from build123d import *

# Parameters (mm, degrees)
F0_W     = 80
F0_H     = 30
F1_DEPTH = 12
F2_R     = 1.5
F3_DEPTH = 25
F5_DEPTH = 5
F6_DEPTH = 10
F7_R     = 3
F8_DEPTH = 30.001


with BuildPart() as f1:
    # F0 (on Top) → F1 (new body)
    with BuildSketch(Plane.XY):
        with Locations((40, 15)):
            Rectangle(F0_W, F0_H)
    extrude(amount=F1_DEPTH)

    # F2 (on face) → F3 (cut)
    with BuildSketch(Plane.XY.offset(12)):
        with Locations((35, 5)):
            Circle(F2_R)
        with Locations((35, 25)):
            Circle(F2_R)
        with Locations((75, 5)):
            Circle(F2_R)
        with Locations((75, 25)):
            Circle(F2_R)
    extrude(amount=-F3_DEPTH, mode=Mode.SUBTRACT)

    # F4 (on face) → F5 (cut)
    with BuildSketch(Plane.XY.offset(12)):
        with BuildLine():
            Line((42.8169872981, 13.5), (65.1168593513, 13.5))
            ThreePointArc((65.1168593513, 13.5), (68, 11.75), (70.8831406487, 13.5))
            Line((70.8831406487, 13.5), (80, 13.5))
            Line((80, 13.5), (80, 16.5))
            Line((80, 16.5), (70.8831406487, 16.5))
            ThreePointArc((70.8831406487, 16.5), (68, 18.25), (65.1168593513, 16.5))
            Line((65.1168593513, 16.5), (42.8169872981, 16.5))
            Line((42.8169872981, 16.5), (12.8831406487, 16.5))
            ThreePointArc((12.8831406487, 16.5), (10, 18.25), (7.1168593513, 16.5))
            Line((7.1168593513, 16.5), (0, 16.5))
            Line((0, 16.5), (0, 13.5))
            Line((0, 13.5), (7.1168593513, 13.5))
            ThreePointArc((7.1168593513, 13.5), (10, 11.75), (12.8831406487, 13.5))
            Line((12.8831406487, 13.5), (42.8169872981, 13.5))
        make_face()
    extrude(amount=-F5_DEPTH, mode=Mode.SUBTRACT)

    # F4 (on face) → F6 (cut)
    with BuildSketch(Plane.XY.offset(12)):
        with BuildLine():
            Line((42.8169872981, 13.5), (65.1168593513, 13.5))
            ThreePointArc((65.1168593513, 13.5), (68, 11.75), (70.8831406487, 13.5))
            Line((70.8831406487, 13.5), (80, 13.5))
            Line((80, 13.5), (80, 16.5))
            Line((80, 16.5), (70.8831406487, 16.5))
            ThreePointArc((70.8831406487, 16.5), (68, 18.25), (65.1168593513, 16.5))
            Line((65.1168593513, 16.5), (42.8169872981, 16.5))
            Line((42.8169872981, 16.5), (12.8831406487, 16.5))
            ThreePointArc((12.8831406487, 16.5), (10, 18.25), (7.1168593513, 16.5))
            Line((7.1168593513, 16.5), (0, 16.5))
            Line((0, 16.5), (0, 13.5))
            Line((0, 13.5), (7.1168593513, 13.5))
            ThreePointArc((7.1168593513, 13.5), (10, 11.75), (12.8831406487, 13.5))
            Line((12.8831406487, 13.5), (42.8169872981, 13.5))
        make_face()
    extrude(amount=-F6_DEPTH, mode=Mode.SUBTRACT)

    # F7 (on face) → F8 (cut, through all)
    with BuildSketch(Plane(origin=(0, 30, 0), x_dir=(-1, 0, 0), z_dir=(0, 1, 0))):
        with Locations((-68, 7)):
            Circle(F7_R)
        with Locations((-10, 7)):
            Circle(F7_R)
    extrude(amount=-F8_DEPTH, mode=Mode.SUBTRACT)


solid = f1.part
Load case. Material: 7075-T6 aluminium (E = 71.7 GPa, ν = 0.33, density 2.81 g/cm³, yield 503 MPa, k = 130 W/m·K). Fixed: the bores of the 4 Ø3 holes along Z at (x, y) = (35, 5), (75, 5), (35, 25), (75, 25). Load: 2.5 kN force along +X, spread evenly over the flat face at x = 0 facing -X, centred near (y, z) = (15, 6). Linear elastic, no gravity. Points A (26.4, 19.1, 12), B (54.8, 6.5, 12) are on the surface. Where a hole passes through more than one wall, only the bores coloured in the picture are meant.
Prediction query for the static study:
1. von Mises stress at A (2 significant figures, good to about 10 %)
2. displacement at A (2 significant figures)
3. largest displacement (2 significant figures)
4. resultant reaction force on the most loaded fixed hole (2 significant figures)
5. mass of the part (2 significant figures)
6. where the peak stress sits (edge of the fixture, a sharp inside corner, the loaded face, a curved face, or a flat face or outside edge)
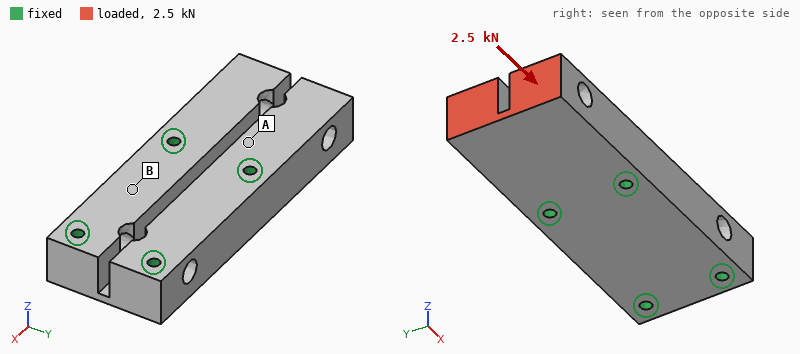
6.3 MPa
1.3 µm
6.2 µm
1.2 kN
69 g
a curved face
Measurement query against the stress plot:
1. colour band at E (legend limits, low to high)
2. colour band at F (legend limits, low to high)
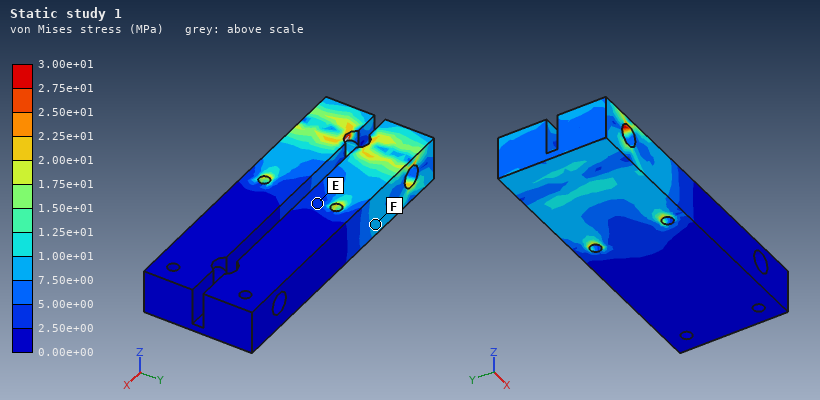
2.50e+00 to 5.00e+00 MPa
7.50e+00 to 1.00e+01 MPa
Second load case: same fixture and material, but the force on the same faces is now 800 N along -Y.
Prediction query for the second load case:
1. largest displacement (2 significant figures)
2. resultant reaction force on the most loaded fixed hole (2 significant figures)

26 µm
1.2 kN
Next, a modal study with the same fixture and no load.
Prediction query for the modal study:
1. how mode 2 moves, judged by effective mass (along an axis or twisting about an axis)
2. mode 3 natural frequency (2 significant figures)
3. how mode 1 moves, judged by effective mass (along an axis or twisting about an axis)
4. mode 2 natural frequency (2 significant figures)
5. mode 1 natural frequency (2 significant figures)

along Y
14 kHz
along Z
9900 Hz
7200 Hz
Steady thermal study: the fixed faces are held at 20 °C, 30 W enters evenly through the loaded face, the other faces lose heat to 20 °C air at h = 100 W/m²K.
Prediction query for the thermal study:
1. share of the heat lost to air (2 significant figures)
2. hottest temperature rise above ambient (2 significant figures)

18 %
27 K
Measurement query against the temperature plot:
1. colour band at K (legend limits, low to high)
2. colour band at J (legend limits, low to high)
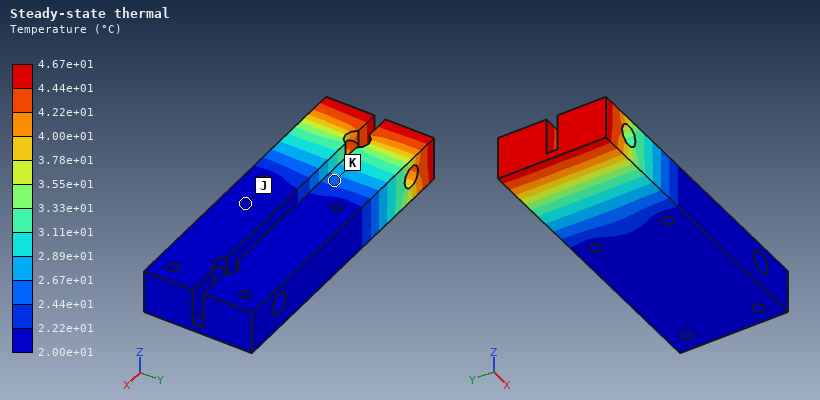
2.44e+01 to 2.67e+01 °C
2.00e+01 to 2.22e+01 °C
